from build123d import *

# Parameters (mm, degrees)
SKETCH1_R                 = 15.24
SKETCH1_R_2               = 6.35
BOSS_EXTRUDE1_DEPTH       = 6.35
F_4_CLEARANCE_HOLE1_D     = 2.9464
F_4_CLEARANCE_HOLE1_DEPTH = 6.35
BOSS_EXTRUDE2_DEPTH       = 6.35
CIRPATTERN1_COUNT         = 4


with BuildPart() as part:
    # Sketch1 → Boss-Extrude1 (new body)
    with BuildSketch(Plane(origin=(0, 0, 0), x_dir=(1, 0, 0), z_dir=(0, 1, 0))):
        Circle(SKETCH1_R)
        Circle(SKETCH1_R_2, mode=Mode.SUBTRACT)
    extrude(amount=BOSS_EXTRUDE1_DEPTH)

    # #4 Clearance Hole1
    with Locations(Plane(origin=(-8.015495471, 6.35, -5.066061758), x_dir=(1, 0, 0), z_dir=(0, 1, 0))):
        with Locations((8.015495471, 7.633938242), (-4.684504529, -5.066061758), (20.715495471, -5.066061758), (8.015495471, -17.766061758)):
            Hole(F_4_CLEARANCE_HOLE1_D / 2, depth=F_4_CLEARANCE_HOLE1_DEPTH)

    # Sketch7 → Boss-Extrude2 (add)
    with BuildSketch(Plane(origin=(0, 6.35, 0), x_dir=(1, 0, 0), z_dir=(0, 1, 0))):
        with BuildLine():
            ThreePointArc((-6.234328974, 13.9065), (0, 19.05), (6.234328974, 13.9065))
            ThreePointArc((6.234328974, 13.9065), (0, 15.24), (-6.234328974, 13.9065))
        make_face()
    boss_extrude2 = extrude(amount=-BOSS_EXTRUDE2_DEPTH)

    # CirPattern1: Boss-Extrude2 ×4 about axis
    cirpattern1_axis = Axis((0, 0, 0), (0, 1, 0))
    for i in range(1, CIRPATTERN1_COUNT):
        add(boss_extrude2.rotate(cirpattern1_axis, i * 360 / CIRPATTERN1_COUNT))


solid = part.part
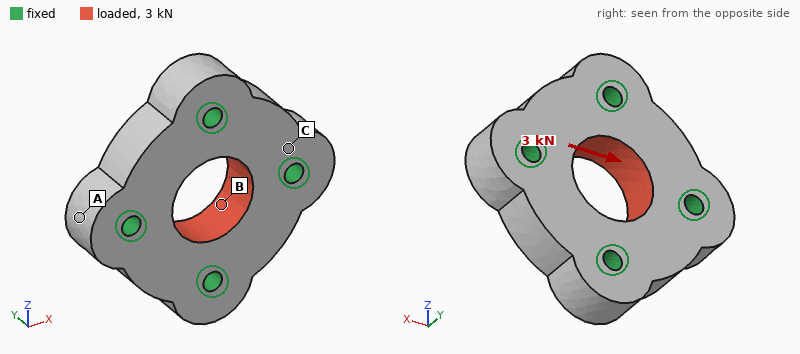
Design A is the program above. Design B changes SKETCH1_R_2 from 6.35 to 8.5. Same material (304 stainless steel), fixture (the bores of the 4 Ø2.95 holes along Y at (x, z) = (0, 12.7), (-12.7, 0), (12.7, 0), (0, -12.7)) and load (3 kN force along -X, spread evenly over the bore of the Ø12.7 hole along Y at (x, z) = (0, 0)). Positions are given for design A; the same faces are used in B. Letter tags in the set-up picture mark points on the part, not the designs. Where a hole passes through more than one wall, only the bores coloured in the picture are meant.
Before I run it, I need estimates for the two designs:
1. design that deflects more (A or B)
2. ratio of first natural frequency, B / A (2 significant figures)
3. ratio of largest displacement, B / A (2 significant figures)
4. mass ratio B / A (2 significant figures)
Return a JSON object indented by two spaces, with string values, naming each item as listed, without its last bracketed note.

{
  "design that deflects more": "A",
  "ratio of first natural frequency, B / A": "1.0",
  "ratio of largest displacement, B / A": "0.91",
  "mass ratio B / A": "0.86"
}
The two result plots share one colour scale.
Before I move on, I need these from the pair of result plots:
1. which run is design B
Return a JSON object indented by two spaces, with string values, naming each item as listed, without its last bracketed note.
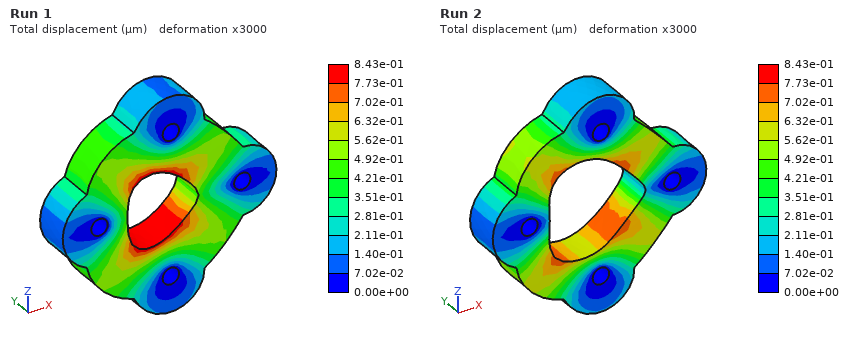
{
  "which run is design B": "Run 2"
}
